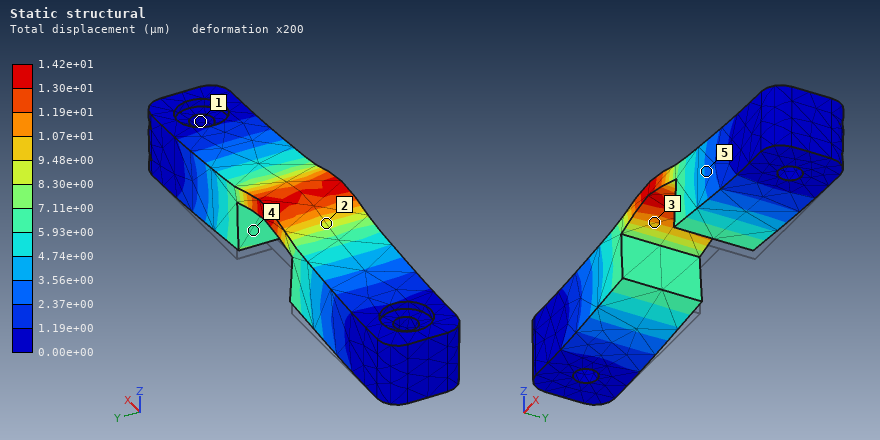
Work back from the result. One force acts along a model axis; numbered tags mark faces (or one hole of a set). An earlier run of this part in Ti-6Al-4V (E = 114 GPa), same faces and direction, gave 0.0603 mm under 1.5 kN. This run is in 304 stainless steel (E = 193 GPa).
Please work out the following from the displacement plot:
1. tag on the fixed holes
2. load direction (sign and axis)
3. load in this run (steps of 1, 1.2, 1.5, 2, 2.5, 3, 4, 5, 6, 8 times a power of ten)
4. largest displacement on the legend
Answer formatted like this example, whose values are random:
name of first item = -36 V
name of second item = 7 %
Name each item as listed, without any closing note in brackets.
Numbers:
tag on the fixed holes = 1
load direction = +Z
load in this run = 600 N
largest displacement on the legend = 1.42e+01 µm
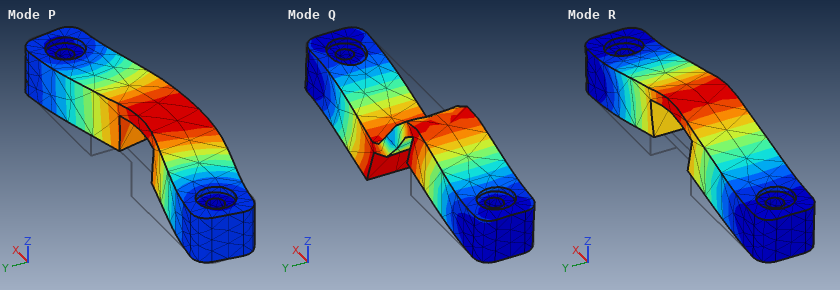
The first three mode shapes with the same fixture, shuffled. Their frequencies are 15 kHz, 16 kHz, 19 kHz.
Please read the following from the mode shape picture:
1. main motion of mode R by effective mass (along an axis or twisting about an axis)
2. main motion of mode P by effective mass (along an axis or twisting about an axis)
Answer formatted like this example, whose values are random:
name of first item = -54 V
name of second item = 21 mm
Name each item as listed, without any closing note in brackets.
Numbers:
main motion of mode R by effective mass = along Z
main motion of mode P by effective mass = along Y
